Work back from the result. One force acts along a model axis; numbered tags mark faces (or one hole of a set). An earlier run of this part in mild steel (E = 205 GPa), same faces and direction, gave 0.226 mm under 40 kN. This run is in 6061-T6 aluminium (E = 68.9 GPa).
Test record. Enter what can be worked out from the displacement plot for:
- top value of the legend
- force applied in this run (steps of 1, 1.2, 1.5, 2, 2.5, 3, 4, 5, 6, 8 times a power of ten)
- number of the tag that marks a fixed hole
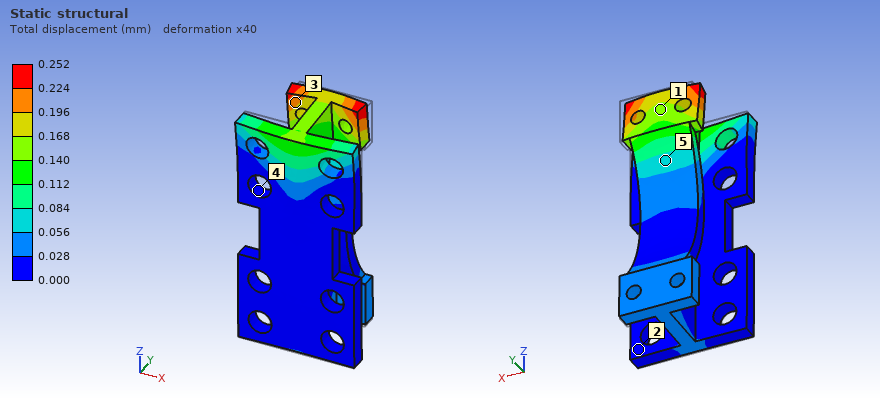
0.252 mm
15 kN
4
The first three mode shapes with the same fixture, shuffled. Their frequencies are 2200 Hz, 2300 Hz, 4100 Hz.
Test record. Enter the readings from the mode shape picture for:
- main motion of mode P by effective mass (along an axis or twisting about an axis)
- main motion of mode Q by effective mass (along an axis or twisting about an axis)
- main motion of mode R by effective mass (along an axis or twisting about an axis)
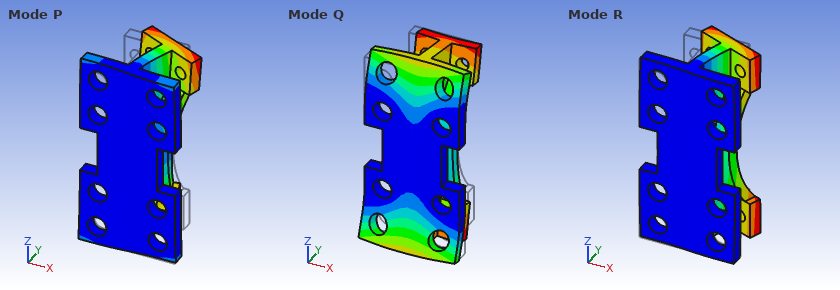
twisting about Y
along Z
along X
